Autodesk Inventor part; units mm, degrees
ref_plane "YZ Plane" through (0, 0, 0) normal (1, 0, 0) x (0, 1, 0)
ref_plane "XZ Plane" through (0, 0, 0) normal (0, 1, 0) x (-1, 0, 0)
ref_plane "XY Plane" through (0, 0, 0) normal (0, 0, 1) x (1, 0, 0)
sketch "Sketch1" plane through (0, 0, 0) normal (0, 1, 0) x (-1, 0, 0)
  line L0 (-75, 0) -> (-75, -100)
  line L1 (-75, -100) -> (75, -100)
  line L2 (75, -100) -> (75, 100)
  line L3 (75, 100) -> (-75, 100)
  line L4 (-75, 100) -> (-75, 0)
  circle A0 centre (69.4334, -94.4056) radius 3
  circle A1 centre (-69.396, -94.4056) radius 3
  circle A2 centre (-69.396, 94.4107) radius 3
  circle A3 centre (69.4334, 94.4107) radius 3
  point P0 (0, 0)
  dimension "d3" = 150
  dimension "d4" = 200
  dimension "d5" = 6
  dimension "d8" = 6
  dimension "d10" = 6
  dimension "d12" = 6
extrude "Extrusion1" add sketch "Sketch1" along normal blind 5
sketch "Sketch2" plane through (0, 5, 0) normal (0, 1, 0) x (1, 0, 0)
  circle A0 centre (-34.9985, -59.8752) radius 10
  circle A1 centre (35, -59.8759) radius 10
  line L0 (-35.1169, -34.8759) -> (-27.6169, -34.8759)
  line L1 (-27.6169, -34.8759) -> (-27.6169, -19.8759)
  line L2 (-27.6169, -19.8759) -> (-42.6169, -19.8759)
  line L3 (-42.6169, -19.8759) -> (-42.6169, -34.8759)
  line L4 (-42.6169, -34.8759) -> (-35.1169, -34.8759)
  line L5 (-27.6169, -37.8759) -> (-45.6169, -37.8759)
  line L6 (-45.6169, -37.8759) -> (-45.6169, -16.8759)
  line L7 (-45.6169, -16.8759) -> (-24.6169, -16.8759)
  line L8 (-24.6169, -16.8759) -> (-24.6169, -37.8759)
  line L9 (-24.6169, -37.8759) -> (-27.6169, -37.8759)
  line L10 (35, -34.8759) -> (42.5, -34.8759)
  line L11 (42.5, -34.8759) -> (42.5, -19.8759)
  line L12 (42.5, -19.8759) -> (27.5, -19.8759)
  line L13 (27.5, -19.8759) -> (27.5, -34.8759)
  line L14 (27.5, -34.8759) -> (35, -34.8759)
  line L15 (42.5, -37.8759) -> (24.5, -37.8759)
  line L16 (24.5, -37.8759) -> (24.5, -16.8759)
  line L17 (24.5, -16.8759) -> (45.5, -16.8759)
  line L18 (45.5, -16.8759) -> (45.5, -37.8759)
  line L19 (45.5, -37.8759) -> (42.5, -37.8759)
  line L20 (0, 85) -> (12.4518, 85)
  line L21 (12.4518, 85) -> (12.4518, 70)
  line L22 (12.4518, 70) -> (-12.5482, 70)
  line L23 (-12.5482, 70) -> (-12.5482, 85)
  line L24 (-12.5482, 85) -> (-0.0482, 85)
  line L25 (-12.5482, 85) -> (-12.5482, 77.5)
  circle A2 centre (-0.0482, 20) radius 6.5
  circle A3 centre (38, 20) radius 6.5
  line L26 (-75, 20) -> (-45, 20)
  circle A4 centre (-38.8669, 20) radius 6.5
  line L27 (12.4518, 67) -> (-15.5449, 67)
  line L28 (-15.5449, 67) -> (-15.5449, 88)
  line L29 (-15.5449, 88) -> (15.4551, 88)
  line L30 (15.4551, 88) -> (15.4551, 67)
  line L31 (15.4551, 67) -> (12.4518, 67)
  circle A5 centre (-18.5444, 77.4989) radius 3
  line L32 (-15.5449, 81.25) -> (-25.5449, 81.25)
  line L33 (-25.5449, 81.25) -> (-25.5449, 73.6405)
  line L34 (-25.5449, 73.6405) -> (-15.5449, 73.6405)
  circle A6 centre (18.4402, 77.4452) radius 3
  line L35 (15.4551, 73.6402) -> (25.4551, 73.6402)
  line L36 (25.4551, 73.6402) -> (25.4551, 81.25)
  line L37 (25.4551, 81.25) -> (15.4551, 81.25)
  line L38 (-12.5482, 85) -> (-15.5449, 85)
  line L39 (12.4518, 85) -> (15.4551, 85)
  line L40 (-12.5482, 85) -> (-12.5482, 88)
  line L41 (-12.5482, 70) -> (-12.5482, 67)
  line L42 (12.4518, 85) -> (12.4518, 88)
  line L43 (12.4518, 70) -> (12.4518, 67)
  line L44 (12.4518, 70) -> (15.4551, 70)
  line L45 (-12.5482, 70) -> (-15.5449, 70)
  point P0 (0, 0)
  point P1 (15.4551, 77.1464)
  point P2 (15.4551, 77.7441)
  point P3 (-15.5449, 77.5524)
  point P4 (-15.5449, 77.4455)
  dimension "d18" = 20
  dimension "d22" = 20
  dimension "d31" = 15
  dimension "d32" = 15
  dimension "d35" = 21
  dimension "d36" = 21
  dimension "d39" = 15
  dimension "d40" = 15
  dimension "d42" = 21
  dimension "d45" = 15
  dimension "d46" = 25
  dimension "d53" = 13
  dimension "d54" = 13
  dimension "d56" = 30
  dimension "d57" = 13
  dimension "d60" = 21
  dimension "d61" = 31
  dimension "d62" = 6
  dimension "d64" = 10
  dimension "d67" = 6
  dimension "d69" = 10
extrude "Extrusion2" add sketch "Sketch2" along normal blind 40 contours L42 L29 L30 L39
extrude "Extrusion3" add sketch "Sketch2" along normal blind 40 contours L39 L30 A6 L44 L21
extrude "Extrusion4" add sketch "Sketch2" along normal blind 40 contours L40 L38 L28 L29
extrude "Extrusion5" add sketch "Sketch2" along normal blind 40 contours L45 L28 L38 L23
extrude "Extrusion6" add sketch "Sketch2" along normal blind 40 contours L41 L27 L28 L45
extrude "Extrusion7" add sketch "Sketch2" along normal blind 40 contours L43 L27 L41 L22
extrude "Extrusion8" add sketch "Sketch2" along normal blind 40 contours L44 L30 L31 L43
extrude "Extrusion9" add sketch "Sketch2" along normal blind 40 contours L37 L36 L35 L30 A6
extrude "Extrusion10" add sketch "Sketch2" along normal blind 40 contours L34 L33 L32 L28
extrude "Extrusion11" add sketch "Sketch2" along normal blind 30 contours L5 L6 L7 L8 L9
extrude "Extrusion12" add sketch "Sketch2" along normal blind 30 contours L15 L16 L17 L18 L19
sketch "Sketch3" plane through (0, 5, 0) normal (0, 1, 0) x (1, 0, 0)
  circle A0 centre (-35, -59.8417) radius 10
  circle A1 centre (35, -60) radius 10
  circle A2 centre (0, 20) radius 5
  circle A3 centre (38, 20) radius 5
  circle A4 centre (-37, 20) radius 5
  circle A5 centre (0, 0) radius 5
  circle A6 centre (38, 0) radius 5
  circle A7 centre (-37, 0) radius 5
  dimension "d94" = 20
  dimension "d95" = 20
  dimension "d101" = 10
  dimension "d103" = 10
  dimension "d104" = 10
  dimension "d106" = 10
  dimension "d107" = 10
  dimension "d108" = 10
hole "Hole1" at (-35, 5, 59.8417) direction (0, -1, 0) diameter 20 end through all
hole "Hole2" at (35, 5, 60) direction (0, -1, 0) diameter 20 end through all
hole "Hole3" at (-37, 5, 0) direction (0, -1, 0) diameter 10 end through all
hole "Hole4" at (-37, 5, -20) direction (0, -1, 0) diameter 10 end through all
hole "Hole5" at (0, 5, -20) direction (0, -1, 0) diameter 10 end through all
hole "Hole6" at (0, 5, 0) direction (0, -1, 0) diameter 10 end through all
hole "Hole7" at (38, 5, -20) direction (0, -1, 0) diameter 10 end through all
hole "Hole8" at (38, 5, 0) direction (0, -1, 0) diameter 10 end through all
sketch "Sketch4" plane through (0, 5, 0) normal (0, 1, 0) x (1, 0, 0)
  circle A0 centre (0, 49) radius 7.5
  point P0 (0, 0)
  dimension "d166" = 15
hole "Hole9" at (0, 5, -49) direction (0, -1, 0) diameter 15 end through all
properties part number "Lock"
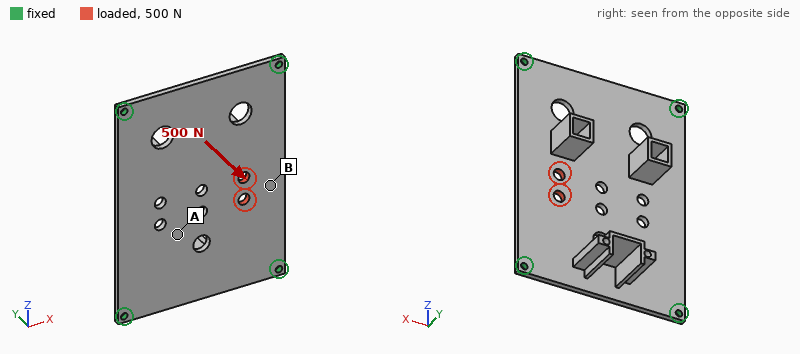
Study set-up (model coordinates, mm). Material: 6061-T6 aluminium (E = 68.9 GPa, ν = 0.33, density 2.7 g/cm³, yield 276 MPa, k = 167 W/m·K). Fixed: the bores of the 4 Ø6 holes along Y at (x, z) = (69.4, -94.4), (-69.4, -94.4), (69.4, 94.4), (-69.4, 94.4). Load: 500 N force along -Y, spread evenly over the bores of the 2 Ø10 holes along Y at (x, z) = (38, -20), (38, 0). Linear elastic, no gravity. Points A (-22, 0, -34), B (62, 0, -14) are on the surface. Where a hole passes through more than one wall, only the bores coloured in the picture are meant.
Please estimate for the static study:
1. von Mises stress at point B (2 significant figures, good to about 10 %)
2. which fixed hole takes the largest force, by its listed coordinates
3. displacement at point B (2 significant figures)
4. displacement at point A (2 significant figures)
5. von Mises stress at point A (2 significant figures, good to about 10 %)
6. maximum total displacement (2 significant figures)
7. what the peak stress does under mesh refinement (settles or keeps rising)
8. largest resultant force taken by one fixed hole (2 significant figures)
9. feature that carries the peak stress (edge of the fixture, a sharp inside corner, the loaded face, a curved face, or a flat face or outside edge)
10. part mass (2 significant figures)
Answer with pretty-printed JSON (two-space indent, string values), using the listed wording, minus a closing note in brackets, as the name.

{
  "von Mises stress at point B": "30 MPa",
  "which fixed hole takes the largest force, by its listed coordinates": "(69.4, -94.4)",
  "displacement at point B": "0.36 mm",
  "displacement at point A": "0.19 mm",
  "von Mises stress at point A": "10.0 MPa",
  "maximum total displacement": "0.37 mm",
  "what the peak stress does under mesh refinement": "keeps rising",
  "largest resultant force taken by one fixed hole": "230 N",
  "feature that carries the peak stress": "edge of the fixture",
  "part mass": "450 g"
}
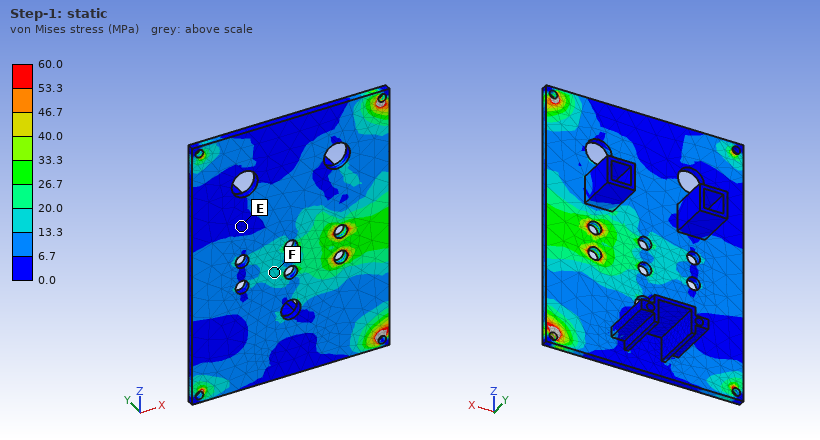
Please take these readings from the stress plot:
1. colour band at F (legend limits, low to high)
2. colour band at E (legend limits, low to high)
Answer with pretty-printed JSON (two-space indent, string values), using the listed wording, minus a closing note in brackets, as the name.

{
  "colour band at F": "13.3 to 20.0 MPa",
  "colour band at E": "0.0 to 6.7 MPa"
}
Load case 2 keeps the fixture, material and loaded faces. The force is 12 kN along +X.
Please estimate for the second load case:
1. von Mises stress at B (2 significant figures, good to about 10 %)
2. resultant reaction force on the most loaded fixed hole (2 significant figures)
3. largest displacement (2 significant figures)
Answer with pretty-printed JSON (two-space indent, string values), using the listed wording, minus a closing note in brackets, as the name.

{
  "von Mises stress at B": "18 MPa",
  "resultant reaction force on the most loaded fixed hole": "4.1 kN",
  "largest displacement": "65 µm"
}
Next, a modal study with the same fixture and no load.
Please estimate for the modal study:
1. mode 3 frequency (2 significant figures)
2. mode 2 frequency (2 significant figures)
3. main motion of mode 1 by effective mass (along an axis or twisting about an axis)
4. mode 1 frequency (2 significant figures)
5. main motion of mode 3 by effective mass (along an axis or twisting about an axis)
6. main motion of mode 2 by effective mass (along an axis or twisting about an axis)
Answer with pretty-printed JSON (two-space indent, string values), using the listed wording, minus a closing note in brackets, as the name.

{
  "mode 3 frequency": "1100 Hz",
  "mode 2 frequency": "860 Hz",
  "main motion of mode 1 by effective mass": "along Y",
  "mode 1 frequency": "480 Hz",
  "main motion of mode 3 by effective mass": "twisting about X",
  "main motion of mode 2 by effective mass": "twisting about Z"
}
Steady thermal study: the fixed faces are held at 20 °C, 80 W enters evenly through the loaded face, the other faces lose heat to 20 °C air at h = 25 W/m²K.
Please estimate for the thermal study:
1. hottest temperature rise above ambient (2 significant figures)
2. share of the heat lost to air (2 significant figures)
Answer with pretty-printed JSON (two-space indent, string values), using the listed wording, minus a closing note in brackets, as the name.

{
  "hottest temperature rise above ambient": "55 K",
  "share of the heat lost to air": "45 %"
}
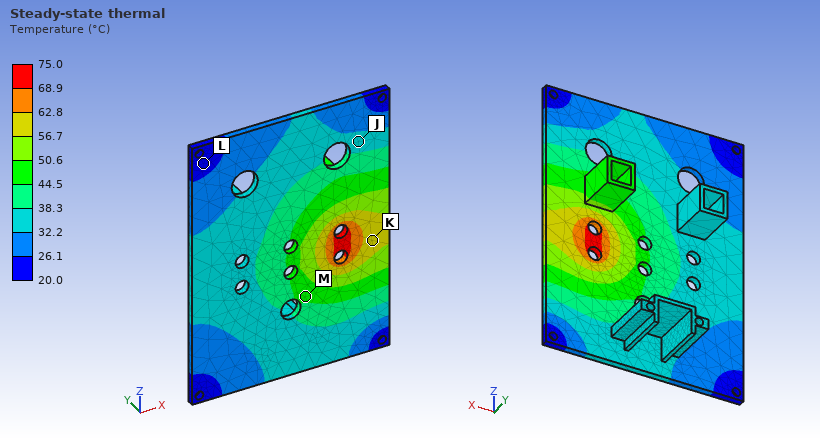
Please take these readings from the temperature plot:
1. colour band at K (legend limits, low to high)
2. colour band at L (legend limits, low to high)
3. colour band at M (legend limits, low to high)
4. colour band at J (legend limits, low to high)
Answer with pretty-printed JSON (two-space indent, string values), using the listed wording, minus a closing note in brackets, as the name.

{
  "colour band at K": "56.7 to 62.8 °C",
  "colour band at L": "20.0 to 26.1 °C",
  "colour band at M": "44.5 to 50.6 °C",
  "colour band at J": "32.2 to 38.3 °C"
}
